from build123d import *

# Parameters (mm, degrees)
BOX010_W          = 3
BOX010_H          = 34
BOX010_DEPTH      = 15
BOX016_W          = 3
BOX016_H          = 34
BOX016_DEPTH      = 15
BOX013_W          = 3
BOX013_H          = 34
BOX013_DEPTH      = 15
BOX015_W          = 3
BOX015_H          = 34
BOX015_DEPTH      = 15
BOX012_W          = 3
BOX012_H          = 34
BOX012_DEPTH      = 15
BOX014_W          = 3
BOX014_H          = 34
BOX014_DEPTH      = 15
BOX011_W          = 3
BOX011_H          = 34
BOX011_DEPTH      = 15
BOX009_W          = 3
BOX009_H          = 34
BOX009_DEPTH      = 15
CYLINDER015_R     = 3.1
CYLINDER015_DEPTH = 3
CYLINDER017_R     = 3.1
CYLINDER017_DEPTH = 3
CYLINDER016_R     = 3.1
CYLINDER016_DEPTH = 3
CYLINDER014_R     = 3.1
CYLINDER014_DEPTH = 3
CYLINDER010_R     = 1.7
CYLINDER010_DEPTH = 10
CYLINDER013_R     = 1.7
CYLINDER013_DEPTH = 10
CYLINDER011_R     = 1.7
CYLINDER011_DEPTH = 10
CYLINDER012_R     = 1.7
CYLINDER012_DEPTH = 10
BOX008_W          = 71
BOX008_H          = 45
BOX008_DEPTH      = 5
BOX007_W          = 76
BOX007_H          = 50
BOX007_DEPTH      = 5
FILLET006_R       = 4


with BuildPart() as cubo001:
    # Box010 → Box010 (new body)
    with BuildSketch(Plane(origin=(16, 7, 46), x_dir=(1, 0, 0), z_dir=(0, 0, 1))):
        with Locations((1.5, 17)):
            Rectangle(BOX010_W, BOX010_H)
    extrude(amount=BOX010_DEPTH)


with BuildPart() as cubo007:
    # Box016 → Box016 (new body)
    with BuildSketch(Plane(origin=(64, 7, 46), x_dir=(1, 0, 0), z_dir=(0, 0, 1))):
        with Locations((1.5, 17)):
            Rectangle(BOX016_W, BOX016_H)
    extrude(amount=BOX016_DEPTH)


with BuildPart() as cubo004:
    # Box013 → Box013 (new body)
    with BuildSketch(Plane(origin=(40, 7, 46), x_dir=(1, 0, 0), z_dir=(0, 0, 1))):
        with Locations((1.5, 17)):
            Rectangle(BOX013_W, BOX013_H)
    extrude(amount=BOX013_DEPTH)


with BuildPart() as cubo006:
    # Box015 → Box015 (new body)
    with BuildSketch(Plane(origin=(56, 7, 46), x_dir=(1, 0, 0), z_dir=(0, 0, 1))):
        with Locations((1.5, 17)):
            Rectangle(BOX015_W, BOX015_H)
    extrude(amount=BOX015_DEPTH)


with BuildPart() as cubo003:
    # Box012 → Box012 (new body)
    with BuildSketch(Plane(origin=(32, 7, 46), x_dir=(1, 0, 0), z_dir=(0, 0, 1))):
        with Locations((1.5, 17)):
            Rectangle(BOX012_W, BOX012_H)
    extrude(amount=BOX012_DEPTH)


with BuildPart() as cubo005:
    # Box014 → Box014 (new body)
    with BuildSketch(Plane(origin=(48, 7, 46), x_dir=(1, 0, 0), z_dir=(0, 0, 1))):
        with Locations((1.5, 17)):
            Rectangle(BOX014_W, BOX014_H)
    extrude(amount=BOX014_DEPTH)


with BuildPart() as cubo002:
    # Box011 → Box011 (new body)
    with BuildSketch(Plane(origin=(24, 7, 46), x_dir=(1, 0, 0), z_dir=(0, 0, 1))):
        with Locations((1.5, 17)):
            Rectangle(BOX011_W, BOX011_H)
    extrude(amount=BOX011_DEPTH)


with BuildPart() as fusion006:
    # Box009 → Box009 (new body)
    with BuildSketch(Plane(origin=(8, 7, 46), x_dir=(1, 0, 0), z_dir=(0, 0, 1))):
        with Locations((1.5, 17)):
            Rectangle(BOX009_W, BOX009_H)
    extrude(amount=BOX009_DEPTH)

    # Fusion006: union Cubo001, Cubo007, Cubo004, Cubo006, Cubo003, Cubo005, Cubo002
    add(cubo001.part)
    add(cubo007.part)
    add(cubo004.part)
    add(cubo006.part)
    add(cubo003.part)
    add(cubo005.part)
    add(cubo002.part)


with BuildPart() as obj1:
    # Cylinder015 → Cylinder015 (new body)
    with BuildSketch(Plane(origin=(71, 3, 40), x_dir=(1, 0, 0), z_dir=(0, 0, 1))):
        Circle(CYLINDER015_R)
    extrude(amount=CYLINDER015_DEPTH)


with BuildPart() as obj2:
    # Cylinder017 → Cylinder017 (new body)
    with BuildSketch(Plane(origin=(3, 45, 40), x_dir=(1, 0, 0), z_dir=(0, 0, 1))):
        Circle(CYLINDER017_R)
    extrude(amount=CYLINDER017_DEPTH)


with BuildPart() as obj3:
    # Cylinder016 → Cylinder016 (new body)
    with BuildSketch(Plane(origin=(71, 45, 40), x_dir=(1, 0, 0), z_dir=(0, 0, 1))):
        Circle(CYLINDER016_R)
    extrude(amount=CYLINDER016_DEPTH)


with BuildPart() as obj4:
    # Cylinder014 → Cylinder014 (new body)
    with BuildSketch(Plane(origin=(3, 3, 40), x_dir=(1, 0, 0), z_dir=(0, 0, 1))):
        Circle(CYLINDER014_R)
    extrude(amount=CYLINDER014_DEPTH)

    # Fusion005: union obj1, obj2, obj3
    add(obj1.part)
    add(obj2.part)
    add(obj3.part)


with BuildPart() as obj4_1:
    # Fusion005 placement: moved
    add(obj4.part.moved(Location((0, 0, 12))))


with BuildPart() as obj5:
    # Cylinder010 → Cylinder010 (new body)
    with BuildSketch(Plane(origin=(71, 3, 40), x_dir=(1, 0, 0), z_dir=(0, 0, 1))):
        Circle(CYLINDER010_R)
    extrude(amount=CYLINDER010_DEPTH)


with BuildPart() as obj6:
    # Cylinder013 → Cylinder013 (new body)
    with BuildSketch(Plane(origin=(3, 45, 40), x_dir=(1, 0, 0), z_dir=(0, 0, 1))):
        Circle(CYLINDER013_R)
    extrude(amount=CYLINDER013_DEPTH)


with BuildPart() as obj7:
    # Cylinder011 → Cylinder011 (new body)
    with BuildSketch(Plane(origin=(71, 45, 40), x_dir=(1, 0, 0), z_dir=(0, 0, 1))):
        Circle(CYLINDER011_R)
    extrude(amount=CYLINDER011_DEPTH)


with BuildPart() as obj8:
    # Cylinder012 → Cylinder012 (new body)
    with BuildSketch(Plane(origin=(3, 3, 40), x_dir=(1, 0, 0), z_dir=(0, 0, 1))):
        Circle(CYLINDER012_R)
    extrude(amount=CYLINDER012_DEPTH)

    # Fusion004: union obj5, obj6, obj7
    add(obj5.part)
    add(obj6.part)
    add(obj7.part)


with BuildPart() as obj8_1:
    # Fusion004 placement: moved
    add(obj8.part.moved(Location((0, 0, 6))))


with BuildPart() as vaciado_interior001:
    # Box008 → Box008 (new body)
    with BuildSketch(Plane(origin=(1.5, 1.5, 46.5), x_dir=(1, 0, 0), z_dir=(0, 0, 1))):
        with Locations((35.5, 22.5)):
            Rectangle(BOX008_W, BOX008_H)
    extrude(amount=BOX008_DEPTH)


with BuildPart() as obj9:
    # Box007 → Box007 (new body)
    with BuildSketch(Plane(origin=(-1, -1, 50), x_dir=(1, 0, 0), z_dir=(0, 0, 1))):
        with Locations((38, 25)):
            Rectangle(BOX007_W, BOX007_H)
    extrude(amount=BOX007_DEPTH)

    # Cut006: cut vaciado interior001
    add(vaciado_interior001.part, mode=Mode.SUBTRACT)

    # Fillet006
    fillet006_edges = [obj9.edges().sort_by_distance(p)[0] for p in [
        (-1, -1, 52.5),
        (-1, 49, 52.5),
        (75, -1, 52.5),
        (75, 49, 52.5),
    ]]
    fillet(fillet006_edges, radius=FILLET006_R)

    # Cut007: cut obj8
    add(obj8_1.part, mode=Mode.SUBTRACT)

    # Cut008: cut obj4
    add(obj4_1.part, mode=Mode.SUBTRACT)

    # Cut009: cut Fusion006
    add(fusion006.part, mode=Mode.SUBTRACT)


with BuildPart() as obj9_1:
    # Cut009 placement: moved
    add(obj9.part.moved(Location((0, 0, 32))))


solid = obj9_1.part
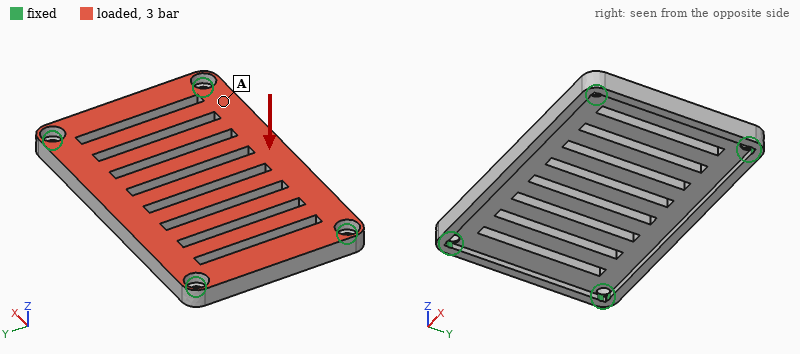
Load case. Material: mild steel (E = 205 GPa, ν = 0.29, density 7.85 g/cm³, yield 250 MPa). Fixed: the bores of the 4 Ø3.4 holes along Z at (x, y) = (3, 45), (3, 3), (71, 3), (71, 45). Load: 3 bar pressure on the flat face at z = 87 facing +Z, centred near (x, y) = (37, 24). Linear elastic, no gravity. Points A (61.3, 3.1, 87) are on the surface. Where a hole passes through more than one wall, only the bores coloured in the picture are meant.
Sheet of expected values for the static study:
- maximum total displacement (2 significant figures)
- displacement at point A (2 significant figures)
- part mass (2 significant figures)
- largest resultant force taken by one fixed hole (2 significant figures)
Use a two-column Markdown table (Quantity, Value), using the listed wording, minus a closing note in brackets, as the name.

| Quantity | Value |
|---|---|
| maximum total displacement | 68 µm |
| displacement at point A | 20 µm |
| part mass | 86 g |
| largest resultant force taken by one fixed hole | 490 N |
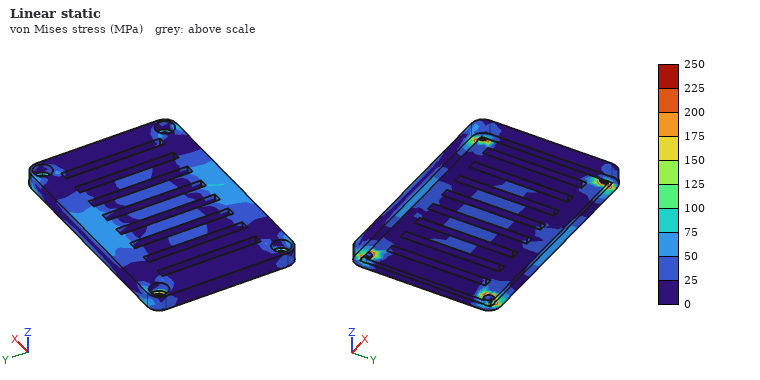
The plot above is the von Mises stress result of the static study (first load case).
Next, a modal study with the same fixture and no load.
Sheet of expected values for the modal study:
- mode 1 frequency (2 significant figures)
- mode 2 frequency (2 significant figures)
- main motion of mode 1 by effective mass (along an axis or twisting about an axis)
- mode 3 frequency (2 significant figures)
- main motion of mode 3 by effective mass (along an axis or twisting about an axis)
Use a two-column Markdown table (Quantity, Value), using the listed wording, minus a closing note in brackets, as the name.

| Quantity | Value |
|---|---|
| mode 1 frequency | 2400 Hz |
| mode 2 frequency | 4100 Hz |
| main motion of mode 1 by effective mass | along Z |
| mode 3 frequency | 5200 Hz |
| main motion of mode 3 by effective mass | twisting about Y |
